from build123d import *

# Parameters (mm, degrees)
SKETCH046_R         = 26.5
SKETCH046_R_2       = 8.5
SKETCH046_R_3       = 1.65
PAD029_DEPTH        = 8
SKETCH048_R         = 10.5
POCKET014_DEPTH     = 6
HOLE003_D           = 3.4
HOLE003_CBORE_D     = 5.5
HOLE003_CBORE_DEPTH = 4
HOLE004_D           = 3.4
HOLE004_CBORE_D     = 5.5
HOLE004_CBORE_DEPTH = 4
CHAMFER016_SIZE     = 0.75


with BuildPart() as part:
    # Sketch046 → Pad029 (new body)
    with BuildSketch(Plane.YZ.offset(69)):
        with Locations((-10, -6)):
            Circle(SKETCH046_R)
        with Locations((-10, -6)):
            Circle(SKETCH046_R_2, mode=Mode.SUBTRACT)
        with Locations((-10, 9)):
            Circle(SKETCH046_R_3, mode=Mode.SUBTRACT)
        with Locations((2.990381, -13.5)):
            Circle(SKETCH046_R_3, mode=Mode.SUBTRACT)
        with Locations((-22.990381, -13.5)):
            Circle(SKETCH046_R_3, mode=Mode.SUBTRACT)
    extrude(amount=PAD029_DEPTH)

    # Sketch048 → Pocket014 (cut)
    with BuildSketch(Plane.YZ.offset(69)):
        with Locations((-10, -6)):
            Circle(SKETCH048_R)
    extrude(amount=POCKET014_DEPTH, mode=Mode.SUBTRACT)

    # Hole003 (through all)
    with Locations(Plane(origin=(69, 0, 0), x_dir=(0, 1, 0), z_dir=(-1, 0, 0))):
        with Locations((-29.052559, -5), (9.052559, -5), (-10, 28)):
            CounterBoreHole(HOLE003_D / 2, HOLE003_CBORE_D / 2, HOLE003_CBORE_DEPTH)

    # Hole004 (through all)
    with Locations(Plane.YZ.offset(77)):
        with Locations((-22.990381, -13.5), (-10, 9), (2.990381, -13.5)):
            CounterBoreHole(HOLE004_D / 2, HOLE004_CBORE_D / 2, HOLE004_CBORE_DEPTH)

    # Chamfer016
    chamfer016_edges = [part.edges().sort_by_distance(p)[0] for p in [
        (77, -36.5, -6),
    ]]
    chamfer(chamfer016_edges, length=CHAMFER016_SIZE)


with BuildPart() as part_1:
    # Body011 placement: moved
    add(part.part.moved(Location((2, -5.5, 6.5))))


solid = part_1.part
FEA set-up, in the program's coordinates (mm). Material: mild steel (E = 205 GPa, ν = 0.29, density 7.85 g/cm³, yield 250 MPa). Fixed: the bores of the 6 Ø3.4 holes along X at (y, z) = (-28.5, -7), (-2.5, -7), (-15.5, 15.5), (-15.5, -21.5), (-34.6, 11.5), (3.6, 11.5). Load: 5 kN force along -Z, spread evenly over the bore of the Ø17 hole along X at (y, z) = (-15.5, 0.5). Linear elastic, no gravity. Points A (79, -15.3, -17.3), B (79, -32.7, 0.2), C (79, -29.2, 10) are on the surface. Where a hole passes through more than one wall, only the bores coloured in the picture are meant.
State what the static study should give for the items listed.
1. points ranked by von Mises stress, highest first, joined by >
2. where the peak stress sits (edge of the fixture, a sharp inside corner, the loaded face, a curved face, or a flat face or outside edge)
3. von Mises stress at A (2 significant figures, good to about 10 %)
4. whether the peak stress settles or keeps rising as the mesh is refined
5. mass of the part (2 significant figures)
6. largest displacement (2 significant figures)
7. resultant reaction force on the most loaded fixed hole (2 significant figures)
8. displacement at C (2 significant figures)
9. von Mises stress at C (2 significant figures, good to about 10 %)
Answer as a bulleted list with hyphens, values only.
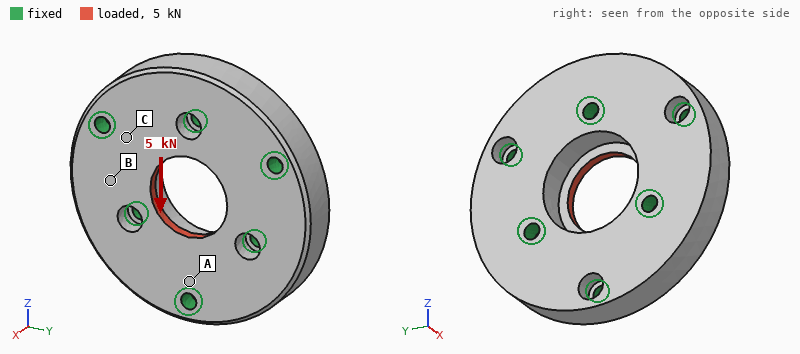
- A > C > B
- edge of the fixture
- 39 MPa
- keeps rising
- 110 g
- 4.2 µm
- 1.0 kN
- 0.66 µm
- 20 MPa
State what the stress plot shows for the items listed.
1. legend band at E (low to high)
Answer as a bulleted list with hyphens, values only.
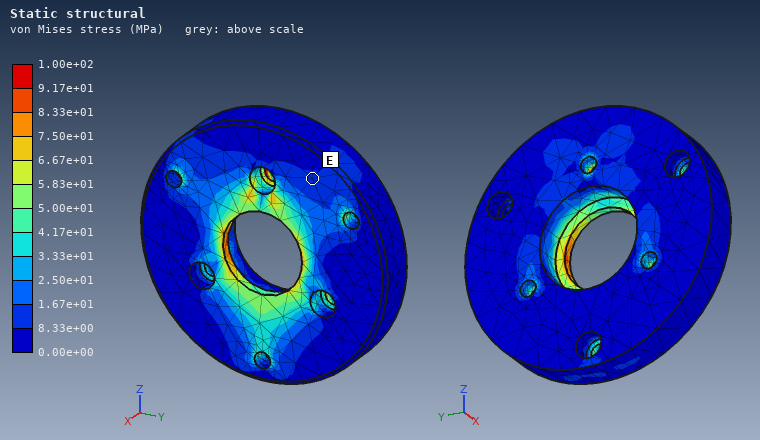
- 8.33e+00 to 1.67e+01 MPa
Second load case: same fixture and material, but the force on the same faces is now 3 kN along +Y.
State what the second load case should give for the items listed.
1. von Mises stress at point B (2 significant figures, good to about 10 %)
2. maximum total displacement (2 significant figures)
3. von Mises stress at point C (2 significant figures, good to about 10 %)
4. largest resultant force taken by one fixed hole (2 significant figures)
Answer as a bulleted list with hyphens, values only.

- 9.6 MPa
- 2.3 µm
- 17 MPa
- 570 N
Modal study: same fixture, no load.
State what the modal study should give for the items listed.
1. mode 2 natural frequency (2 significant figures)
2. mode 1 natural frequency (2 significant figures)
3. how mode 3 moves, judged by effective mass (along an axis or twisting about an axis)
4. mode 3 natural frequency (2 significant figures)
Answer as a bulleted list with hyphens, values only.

- 25 kHz
- 25 kHz
- along X
- 27 kHz
